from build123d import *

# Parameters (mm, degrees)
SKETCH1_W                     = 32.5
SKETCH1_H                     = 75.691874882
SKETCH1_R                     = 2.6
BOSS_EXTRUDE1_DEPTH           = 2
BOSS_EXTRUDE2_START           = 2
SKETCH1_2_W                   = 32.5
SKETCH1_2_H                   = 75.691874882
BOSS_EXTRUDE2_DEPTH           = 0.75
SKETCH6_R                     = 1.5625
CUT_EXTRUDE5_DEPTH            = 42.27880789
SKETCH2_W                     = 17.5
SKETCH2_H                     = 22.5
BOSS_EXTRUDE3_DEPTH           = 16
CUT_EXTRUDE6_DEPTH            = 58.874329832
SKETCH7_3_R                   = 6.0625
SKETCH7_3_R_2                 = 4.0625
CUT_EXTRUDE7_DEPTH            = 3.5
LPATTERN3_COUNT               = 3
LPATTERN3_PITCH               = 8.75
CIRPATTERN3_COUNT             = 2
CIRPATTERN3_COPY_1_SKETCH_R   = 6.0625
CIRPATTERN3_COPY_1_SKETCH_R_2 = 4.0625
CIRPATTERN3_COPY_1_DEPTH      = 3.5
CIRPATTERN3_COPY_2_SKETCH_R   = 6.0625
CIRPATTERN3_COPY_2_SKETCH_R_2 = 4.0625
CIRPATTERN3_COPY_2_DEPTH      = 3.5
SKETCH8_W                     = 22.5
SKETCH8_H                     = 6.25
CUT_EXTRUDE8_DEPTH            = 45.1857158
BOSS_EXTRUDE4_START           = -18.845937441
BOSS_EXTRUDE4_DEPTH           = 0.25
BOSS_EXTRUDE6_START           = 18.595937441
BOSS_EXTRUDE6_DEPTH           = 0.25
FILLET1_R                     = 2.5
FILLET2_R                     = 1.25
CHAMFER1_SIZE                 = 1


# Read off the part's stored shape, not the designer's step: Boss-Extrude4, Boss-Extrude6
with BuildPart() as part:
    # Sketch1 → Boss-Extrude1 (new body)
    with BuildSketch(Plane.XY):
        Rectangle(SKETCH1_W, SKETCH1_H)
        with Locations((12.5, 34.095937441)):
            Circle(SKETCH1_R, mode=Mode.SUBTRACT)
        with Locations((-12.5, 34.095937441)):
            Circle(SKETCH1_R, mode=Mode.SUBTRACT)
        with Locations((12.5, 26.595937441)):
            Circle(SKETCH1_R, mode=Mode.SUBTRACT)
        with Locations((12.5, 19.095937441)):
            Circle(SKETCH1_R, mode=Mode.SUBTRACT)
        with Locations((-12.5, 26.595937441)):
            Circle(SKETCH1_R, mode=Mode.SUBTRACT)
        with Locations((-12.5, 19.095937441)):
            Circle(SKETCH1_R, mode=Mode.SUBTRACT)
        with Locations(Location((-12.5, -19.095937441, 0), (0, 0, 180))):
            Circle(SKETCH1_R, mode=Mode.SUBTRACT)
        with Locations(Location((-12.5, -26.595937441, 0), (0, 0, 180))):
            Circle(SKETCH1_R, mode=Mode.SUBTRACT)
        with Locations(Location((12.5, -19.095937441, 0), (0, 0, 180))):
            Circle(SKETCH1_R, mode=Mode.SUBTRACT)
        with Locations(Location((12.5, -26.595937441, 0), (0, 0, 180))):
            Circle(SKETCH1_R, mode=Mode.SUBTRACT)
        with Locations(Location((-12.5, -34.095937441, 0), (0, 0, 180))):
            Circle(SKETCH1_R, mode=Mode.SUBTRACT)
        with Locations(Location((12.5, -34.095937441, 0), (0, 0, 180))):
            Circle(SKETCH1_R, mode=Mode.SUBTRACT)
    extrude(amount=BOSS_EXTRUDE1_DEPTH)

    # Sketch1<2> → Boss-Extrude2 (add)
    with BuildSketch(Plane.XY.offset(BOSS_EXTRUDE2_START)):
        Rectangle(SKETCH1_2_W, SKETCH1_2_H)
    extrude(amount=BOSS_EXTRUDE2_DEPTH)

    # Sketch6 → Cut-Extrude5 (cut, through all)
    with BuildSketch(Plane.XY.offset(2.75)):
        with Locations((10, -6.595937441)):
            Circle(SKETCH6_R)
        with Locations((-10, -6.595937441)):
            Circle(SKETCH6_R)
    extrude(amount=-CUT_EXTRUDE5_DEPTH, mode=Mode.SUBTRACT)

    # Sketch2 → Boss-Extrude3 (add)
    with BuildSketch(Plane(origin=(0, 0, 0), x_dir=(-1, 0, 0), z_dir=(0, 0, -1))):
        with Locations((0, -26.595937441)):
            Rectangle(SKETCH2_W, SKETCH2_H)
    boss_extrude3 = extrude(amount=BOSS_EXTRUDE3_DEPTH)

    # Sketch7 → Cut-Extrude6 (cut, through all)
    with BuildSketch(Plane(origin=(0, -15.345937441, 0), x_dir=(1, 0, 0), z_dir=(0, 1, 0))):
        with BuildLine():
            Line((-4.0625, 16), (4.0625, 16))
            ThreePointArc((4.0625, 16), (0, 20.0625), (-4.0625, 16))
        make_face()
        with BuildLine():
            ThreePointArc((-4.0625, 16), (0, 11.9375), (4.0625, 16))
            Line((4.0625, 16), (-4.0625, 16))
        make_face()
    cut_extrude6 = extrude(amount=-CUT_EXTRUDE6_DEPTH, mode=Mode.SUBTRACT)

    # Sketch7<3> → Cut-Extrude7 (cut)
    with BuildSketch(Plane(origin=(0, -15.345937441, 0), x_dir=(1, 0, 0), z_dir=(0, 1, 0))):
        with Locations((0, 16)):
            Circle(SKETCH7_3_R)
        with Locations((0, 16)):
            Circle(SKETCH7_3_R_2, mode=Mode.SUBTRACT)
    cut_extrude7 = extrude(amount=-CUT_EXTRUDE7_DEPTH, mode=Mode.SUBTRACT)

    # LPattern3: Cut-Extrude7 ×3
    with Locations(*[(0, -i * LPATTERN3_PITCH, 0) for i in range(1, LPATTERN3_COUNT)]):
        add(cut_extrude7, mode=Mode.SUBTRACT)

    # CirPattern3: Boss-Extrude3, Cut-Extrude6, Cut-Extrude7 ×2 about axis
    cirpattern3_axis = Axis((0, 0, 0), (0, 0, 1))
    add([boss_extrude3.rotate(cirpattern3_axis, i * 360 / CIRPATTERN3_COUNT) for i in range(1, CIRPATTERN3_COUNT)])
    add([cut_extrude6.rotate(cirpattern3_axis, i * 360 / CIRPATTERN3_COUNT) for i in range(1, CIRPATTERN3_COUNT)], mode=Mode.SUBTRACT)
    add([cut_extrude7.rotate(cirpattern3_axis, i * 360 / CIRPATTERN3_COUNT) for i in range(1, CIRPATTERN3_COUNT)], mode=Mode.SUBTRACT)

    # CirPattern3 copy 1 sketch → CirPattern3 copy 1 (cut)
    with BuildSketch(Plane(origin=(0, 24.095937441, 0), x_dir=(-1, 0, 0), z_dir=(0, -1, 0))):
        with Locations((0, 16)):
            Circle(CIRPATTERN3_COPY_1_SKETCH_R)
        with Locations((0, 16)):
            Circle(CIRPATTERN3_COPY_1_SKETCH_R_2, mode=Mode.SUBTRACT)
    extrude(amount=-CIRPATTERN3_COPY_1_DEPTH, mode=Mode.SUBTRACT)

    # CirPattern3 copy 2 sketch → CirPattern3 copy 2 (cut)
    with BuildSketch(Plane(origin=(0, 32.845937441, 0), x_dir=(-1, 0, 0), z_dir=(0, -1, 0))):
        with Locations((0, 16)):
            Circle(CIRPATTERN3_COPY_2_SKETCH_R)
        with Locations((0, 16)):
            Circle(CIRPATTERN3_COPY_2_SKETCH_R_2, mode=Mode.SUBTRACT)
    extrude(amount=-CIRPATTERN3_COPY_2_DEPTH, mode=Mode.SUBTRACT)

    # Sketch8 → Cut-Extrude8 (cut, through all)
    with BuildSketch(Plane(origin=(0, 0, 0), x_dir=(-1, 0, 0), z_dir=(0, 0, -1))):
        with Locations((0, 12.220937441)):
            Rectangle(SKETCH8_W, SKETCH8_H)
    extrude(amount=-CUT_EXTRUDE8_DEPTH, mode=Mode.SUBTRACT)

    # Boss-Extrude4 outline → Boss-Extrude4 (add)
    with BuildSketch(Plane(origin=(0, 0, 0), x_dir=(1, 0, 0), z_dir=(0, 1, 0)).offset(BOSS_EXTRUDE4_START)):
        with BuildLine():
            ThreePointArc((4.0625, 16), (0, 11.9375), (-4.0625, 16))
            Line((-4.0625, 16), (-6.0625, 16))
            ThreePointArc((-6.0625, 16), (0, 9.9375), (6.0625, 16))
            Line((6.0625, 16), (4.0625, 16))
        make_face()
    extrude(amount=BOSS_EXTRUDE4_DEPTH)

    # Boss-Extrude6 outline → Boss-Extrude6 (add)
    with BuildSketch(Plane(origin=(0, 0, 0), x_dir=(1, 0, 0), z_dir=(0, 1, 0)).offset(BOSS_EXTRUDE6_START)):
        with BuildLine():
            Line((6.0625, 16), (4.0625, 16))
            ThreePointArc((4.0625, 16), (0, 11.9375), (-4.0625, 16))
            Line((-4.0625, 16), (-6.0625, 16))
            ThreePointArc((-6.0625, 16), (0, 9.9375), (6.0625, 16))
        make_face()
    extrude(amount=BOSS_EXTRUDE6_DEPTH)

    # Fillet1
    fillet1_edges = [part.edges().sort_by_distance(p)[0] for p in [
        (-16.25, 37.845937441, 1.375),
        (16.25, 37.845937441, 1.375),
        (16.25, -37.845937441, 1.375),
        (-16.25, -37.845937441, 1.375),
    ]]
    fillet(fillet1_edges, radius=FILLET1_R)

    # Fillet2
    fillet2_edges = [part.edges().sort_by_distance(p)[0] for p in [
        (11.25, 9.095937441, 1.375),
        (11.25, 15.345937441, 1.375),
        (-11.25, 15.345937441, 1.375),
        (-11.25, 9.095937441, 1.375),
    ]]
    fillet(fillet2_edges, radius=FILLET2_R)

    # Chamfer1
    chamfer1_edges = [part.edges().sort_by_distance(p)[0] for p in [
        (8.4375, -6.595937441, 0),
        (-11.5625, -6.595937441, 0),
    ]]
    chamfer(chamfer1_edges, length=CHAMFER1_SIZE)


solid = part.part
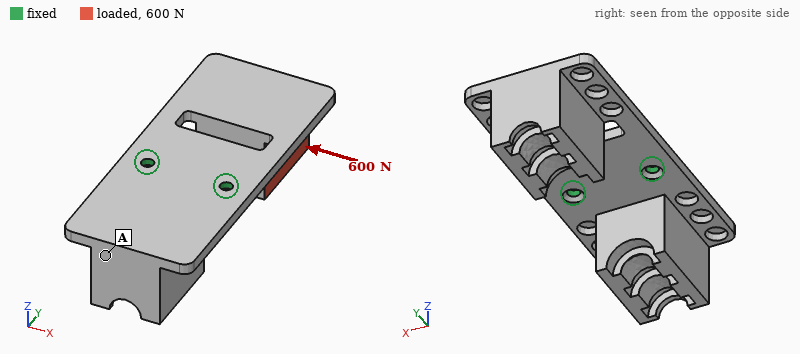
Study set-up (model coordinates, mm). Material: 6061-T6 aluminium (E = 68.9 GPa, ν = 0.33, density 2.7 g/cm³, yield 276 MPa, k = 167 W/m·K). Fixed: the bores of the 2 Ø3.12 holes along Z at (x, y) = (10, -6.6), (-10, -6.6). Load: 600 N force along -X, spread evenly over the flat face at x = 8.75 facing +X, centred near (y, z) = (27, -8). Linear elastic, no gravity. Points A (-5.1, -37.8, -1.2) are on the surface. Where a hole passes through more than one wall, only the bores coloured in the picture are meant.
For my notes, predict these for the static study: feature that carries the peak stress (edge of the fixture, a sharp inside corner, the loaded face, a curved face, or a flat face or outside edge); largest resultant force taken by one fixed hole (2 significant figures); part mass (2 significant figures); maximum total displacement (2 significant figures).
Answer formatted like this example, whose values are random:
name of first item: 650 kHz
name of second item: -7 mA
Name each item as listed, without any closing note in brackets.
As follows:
feature that carries the peak stress: a curved face
largest resultant force taken by one fixed hole: 1.0 kN
part mass: 45 g
maximum total displacement: 0.49 mm
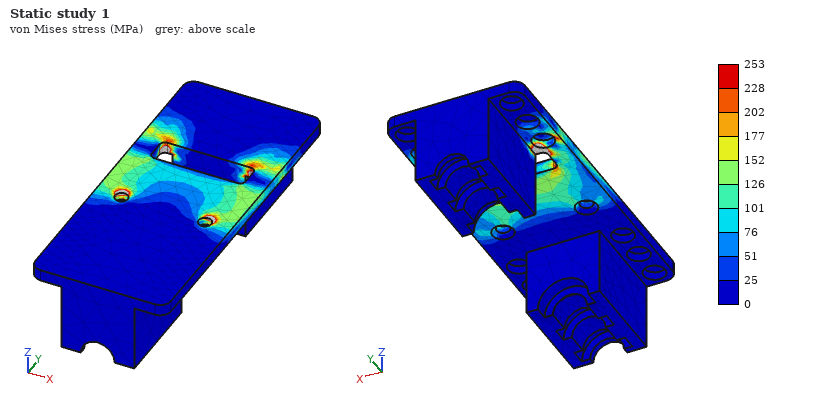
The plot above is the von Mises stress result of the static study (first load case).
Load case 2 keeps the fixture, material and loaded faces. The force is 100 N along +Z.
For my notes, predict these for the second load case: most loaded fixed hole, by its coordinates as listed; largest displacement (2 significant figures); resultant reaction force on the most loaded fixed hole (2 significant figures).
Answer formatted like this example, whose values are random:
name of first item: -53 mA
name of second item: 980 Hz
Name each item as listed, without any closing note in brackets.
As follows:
most loaded fixed hole, by its coordinates as listed: (10, -6.6)
largest displacement: 0.99 mm
resultant reaction force on the most loaded fixed hole: 92 N
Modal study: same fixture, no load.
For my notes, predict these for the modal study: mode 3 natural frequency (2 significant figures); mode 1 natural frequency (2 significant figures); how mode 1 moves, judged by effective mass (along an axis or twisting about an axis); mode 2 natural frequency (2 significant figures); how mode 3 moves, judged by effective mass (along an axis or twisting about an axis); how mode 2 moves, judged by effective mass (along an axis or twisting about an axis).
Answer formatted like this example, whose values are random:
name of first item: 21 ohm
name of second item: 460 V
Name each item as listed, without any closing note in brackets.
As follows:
mode 3 natural frequency: 1700 Hz
mode 1 natural frequency: 430 Hz
how mode 1 moves, judged by effective mass: along Z
mode 2 natural frequency: 1100 Hz
how mode 3 moves, judged by effective mass: along X
how mode 2 moves, judged by effective mass: along Z
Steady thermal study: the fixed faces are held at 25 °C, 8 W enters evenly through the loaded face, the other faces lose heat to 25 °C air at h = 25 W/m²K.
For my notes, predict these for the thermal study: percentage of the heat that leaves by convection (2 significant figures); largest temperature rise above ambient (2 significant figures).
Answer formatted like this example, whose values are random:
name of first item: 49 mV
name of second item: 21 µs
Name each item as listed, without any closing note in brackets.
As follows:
percentage of the heat that leaves by convection: 28 %
largest temperature rise above ambient: 29 K
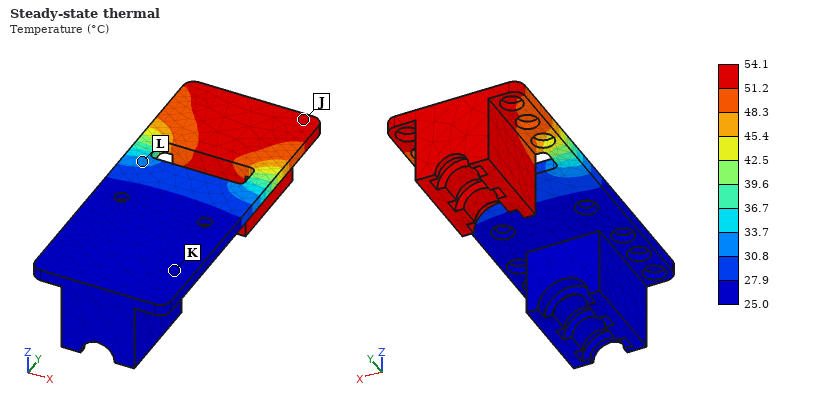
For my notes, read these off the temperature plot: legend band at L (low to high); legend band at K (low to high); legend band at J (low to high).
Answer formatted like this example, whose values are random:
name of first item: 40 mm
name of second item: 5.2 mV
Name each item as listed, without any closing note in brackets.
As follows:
legend band at L: 30.8 to 33.7 °C
legend band at K: 25.0 to 27.9 °C
legend band at J: 51.2 to 54.1 °C
